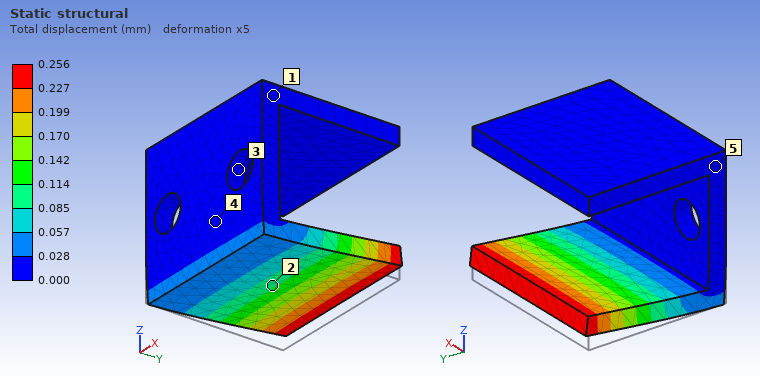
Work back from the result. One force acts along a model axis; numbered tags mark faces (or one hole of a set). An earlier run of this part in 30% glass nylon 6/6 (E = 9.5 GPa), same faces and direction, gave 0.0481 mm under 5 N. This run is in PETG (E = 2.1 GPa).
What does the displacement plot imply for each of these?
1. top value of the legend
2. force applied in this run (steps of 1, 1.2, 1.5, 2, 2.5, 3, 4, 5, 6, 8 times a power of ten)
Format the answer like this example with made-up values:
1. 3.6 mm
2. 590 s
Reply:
1. 0.256 mm
2. 6 N
